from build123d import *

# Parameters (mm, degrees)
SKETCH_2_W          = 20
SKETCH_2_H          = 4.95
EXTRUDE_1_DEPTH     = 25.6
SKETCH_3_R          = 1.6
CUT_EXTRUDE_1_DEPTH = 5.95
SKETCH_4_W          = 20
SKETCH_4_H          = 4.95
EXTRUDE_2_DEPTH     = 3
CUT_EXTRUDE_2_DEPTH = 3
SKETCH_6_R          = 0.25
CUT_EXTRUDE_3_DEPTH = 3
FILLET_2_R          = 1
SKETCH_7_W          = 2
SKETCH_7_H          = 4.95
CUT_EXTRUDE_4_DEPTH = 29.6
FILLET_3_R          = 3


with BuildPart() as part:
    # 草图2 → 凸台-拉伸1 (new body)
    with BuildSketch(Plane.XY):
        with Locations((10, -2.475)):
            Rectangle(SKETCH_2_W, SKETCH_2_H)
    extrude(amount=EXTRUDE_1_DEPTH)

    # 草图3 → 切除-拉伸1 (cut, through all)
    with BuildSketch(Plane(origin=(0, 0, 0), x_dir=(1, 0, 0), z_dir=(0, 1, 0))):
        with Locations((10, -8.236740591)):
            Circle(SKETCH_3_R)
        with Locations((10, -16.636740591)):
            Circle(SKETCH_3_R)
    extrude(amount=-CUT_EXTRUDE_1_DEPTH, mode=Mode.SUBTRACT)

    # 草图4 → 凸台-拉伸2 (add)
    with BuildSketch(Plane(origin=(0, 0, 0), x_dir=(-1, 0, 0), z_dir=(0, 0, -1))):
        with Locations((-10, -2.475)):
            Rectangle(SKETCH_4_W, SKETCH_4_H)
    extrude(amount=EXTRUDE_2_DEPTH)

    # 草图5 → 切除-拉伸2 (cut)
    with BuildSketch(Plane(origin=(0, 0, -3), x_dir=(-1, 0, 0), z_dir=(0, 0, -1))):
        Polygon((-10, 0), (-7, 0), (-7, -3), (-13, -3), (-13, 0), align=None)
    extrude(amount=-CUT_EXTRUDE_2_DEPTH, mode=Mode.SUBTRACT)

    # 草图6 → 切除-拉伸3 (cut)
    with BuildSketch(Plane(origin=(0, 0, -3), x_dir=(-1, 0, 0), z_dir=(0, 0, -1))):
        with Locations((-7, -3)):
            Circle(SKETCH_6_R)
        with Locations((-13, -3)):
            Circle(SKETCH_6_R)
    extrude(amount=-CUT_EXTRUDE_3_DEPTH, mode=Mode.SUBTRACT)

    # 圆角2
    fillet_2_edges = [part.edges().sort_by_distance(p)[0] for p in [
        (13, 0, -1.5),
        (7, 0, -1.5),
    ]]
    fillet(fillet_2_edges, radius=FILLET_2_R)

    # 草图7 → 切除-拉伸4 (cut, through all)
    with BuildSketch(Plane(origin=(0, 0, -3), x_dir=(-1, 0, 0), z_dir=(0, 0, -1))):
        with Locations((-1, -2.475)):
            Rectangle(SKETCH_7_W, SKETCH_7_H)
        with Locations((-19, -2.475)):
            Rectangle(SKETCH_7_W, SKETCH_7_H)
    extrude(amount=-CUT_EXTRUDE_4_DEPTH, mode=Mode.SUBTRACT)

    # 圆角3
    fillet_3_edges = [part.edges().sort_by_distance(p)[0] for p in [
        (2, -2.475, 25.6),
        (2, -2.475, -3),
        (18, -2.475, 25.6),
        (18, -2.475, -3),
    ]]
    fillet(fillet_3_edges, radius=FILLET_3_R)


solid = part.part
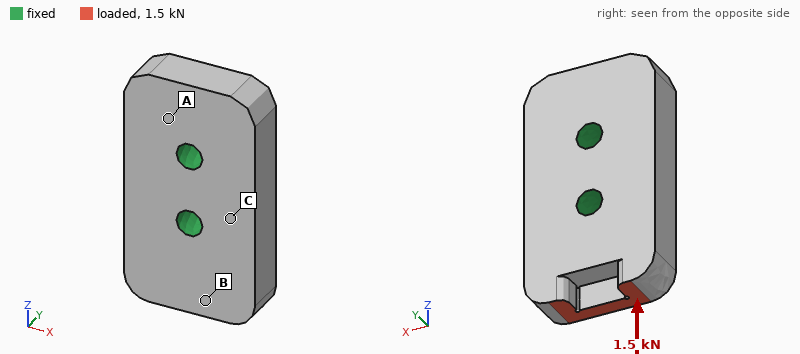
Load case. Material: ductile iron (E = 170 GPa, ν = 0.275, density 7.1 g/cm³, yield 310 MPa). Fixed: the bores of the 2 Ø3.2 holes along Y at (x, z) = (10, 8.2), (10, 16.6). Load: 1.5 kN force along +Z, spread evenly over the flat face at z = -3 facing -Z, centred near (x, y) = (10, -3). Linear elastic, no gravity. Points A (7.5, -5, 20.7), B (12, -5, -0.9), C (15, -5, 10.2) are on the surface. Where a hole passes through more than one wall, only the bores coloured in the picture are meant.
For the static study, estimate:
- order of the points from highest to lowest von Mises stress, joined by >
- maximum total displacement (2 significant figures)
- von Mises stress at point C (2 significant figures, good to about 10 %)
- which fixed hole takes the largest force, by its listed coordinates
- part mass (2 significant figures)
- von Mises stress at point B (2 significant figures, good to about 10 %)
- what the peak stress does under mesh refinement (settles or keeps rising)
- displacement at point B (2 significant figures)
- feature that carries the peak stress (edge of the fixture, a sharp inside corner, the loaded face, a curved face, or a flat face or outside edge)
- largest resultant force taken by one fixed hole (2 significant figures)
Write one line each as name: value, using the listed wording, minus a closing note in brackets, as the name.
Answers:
order of the points from highest to lowest von Mises stress, joined by >: B > C > A
maximum total displacement: 3.9 µm
von Mises stress at point C: 14 MPa
which fixed hole takes the largest force, by its listed coordinates: (10, 8.2)
part mass: 15 g
von Mises stress at point B: 47 MPa
what the peak stress does under mesh refinement: keeps rising
displacement at point B: 3.0 µm
feature that carries the peak stress: a sharp inside corner
largest resultant force taken by one fixed hole: 1.2 kN
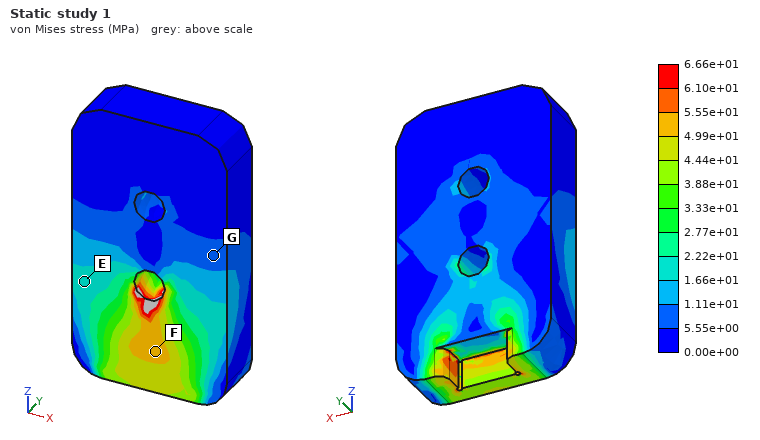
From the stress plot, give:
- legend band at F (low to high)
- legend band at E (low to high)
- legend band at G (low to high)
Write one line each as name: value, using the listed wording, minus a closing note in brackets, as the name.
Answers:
legend band at F: 4.99e+01 to 5.55e+01 MPa
legend band at E: 1.66e+01 to 2.22e+01 MPa
legend band at G: 5.55e+00 to 1.11e+01 MPa
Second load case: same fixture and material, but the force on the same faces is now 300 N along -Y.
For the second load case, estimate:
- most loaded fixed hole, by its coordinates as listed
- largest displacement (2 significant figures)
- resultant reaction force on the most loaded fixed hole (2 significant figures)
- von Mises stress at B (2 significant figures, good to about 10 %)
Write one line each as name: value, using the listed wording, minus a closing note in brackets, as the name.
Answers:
most loaded fixed hole, by its coordinates as listed: (10, 8.2)
largest displacement: 8.6 µm
resultant reaction force on the most loaded fixed hole: 410 N
von Mises stress at B: 36 MPa
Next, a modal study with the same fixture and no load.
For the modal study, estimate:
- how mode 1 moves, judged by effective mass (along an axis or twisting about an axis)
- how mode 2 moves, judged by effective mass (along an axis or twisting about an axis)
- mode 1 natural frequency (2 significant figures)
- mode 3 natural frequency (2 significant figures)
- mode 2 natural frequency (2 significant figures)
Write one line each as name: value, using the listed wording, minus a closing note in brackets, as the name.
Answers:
how mode 1 moves, judged by effective mass: along Y
how mode 2 moves, judged by effective mass: twisting about Z
mode 1 natural frequency: 29 kHz
mode 3 natural frequency: 38 kHz
mode 2 natural frequency: 34 kHz
